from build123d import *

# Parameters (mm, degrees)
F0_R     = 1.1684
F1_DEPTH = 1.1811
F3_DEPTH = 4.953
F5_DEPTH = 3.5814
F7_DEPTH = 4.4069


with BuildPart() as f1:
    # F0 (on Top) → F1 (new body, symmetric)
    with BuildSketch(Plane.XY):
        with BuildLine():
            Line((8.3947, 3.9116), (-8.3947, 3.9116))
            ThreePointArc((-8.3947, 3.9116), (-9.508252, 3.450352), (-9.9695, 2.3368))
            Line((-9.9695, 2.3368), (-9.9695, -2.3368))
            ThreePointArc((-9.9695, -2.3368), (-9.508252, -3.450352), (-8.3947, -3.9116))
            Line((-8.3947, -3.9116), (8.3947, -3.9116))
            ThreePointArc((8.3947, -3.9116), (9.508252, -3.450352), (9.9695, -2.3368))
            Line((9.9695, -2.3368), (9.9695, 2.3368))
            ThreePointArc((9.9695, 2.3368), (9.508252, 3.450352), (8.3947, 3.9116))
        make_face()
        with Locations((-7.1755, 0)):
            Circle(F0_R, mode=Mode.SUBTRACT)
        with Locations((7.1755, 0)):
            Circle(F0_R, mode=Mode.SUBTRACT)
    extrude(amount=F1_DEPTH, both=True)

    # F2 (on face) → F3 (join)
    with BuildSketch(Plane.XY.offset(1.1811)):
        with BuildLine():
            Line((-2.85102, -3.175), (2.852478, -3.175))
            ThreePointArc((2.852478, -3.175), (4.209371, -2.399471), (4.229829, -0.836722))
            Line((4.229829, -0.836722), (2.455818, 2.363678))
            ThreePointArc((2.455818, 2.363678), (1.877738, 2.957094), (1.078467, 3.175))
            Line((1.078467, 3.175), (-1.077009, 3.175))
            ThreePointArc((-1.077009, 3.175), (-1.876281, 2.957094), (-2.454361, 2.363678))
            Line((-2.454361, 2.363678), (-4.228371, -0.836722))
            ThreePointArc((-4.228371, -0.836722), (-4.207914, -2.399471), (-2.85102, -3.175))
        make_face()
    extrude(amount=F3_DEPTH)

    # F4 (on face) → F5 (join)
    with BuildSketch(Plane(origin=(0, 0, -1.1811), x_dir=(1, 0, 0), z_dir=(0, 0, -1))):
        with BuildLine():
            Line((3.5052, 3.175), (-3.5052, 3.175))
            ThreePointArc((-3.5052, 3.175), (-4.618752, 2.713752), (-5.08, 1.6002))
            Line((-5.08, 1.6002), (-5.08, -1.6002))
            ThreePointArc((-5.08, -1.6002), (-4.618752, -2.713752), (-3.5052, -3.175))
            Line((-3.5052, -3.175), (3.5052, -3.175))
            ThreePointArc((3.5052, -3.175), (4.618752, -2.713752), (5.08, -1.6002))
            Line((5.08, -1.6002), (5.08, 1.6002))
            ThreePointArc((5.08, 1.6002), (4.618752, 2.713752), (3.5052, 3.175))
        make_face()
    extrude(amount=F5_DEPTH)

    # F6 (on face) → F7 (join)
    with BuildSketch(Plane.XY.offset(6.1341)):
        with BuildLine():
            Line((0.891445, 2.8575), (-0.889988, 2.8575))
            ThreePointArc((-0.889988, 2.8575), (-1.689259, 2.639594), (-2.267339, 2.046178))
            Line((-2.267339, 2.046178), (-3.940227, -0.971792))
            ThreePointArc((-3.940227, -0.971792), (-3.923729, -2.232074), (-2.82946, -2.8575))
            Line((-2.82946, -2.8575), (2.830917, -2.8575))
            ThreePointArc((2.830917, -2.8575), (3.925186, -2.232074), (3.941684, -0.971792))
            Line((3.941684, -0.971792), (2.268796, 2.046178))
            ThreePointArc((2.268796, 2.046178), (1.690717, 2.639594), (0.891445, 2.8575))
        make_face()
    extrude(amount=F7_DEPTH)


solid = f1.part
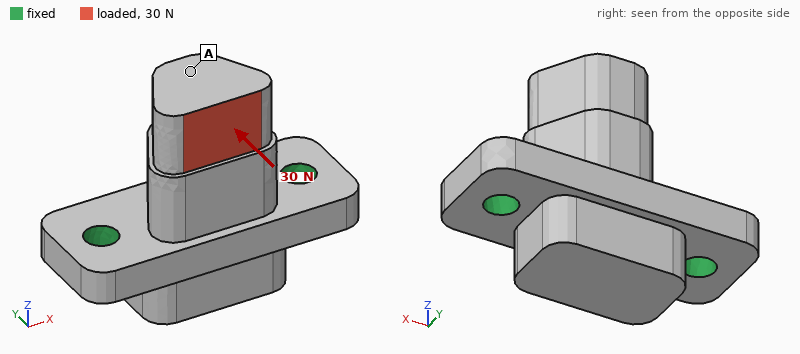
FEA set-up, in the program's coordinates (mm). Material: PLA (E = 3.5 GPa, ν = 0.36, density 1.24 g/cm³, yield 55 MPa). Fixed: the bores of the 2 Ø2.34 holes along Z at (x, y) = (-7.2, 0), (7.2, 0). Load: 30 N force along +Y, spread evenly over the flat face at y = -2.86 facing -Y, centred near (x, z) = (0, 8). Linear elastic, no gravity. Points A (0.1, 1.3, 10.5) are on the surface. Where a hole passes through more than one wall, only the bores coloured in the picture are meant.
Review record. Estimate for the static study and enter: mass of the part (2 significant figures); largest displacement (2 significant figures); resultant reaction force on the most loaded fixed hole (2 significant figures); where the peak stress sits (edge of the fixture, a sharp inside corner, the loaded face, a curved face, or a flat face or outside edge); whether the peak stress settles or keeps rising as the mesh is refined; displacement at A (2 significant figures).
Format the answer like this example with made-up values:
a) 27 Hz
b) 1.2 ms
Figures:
a) 1.2 g
b) 0.11 mm
c) 15 N
d) edge of the fixture
e) keeps rising
f) 0.11 mm
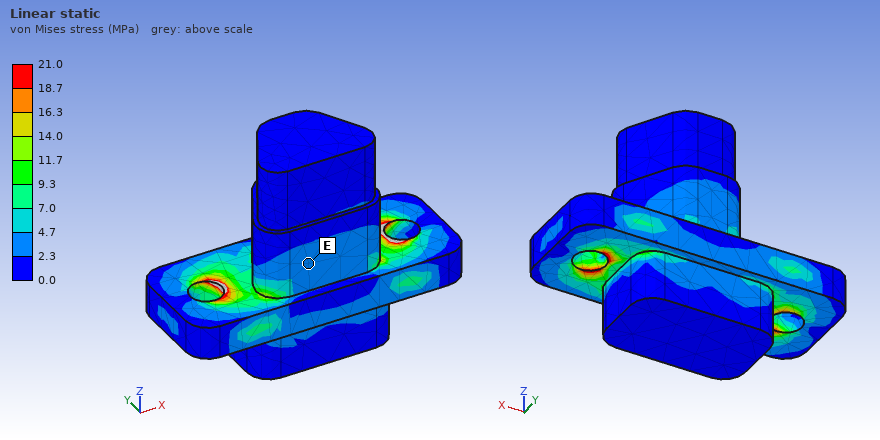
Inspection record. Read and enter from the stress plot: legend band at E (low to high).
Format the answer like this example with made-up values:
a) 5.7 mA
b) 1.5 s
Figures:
a) 2.3 to 4.7 MPa
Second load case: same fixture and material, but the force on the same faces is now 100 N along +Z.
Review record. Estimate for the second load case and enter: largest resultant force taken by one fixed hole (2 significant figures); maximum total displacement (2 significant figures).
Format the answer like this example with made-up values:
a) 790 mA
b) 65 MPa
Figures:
a) 50 N
b) 0.13 mm
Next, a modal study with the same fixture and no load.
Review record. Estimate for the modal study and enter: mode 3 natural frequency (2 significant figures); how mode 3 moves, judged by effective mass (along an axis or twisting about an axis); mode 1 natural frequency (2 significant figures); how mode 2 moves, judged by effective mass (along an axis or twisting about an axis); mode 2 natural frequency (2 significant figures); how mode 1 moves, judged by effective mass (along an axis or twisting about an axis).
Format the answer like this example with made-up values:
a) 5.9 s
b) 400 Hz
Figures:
a) 14 kHz
b) along Z
c) 5400 Hz
d) along X
e) 11 kHz
f) along Y
